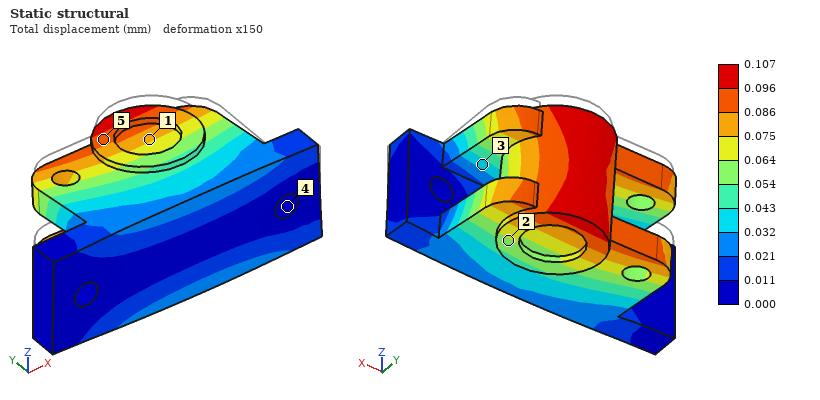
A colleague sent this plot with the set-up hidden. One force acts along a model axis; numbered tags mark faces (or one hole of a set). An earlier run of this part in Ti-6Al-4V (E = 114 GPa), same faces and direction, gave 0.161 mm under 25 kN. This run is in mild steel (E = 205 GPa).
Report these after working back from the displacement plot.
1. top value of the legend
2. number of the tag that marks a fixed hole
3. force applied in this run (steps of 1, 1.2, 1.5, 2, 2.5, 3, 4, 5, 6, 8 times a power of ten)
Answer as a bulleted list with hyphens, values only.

- 0.107 mm
- 4
- 30 kN
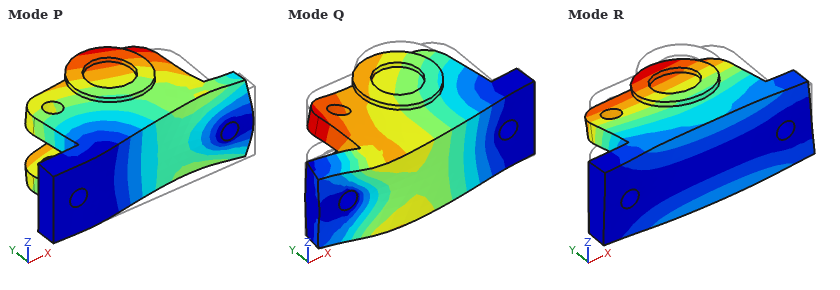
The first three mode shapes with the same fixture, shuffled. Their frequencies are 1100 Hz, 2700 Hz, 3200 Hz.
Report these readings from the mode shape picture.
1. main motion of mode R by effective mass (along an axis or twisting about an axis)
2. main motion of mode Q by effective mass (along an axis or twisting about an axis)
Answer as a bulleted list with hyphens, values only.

- along Z
- along Y
